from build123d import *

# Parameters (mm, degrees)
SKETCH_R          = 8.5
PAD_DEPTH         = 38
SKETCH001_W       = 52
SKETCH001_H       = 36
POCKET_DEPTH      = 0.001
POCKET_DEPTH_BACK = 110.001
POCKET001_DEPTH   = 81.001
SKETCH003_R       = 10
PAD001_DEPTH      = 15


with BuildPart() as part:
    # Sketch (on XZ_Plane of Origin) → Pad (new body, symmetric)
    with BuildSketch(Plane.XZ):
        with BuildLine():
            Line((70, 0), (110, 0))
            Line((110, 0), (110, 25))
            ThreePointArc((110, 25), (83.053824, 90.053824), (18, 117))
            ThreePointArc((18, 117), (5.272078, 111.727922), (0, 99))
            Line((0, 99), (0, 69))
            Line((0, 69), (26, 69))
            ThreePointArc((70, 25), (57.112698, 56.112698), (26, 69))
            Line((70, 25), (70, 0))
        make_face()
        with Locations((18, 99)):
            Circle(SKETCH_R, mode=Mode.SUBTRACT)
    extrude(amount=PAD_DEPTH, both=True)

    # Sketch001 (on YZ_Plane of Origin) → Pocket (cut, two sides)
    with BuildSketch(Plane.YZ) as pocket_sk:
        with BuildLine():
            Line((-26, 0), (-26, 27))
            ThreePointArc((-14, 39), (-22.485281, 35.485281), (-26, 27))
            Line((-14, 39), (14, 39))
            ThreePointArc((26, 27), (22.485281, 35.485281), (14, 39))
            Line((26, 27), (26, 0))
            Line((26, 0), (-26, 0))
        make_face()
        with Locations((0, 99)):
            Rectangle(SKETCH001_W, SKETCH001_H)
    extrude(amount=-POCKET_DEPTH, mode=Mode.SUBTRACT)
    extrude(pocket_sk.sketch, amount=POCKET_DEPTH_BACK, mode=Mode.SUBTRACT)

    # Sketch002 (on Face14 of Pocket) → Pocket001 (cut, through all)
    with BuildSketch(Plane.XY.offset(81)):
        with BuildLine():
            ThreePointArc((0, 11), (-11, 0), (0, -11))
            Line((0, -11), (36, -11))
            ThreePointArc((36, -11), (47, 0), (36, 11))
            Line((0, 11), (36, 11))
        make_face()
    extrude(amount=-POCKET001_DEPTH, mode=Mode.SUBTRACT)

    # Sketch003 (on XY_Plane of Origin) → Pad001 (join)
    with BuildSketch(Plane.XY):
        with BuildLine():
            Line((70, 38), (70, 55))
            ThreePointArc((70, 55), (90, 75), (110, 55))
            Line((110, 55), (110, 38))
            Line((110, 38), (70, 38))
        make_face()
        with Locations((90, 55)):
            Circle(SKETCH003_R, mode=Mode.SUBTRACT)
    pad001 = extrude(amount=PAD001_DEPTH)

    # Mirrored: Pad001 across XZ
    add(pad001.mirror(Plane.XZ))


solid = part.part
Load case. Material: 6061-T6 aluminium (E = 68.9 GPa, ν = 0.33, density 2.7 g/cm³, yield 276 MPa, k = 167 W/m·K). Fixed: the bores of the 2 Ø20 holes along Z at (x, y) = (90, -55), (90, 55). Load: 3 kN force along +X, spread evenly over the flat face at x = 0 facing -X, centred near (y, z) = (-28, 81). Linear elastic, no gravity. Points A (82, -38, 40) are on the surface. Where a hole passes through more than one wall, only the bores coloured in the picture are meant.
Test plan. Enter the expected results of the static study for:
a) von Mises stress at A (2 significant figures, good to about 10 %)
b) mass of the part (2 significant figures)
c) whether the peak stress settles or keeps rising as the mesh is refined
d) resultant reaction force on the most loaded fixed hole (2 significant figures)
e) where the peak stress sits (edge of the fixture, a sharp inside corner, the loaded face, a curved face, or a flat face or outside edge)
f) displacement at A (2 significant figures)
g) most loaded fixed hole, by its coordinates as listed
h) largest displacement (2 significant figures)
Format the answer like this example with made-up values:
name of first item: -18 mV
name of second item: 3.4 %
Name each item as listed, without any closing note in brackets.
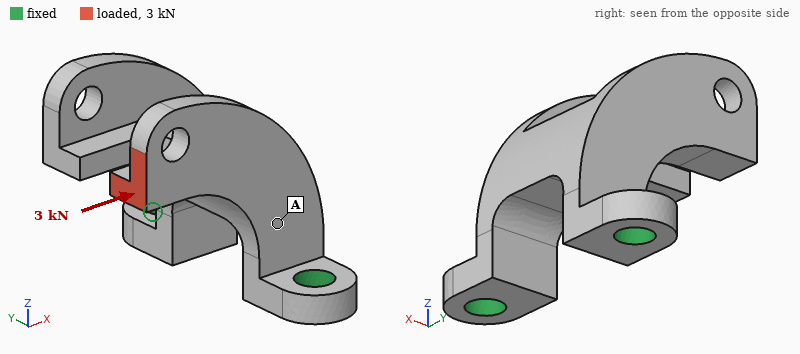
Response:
von Mises stress at A: 12 MPa
mass of the part: 830 g
whether the peak stress settles or keeps rising as the mesh is refined: keeps rising
resultant reaction force on the most loaded fixed hole: 2.5 kN
where the peak stress sits: edge of the fixture
displacement at A: 0.067 mm
most loaded fixed hole, by its coordinates as listed: (90, -55)
largest displacement: 0.28 mm
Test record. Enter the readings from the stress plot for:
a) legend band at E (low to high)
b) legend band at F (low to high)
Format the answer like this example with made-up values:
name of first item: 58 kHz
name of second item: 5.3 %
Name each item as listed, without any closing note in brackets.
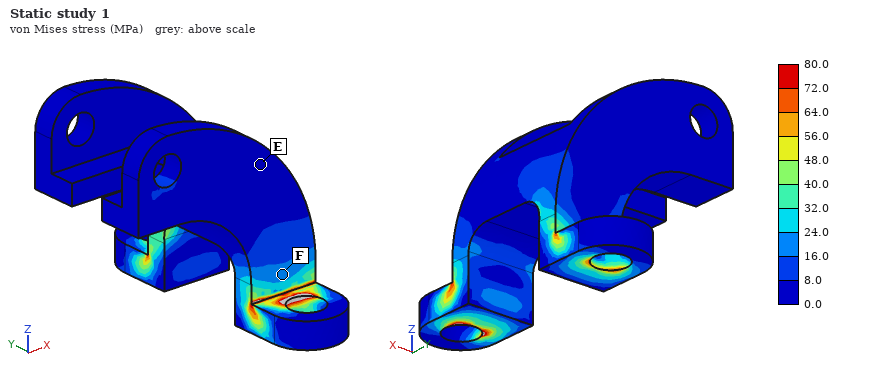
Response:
legend band at E: 0.0 to 8.0 MPa
legend band at F: 16.0 to 24.0 MPa
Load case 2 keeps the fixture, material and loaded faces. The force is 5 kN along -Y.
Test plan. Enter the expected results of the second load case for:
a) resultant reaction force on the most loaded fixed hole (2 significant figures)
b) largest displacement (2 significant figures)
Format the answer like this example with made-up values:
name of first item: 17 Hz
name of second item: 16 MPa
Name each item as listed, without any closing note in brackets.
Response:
resultant reaction force on the most loaded fixed hole: 7.4 kN
largest displacement: 0.40 mm
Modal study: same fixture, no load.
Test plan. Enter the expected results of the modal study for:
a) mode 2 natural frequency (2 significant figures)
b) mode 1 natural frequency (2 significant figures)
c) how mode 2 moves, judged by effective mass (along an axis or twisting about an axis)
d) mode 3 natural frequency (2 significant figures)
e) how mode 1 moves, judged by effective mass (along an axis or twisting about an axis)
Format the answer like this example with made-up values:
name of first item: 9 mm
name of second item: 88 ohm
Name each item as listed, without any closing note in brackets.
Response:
mode 2 natural frequency: 1800 Hz
mode 1 natural frequency: 890 Hz
how mode 2 moves, judged by effective mass: along Y
mode 3 natural frequency: 3000 Hz
how mode 1 moves, judged by effective mass: along X
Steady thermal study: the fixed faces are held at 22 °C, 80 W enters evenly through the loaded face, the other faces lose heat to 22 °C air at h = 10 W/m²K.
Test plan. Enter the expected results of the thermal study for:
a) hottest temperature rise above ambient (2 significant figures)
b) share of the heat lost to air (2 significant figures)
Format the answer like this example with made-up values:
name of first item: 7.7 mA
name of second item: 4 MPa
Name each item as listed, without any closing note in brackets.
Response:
hottest temperature rise above ambient: 73 K
share of the heat lost to air: 13 %
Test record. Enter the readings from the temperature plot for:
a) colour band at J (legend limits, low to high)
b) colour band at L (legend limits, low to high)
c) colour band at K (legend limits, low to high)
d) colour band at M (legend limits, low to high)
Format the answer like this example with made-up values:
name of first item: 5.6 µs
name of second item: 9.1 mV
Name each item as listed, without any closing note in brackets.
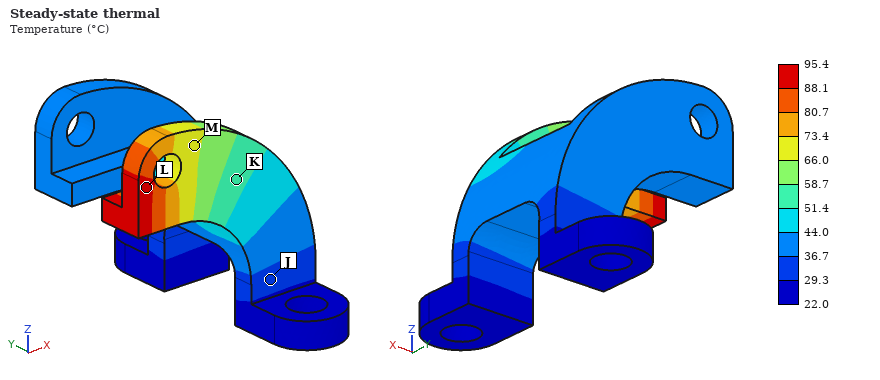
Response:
colour band at J: 29.3 to 36.7 °C
colour band at L: 88.1 to 95.4 °C
colour band at K: 51.4 to 58.7 °C
colour band at M: 66.0 to 73.4 °C
